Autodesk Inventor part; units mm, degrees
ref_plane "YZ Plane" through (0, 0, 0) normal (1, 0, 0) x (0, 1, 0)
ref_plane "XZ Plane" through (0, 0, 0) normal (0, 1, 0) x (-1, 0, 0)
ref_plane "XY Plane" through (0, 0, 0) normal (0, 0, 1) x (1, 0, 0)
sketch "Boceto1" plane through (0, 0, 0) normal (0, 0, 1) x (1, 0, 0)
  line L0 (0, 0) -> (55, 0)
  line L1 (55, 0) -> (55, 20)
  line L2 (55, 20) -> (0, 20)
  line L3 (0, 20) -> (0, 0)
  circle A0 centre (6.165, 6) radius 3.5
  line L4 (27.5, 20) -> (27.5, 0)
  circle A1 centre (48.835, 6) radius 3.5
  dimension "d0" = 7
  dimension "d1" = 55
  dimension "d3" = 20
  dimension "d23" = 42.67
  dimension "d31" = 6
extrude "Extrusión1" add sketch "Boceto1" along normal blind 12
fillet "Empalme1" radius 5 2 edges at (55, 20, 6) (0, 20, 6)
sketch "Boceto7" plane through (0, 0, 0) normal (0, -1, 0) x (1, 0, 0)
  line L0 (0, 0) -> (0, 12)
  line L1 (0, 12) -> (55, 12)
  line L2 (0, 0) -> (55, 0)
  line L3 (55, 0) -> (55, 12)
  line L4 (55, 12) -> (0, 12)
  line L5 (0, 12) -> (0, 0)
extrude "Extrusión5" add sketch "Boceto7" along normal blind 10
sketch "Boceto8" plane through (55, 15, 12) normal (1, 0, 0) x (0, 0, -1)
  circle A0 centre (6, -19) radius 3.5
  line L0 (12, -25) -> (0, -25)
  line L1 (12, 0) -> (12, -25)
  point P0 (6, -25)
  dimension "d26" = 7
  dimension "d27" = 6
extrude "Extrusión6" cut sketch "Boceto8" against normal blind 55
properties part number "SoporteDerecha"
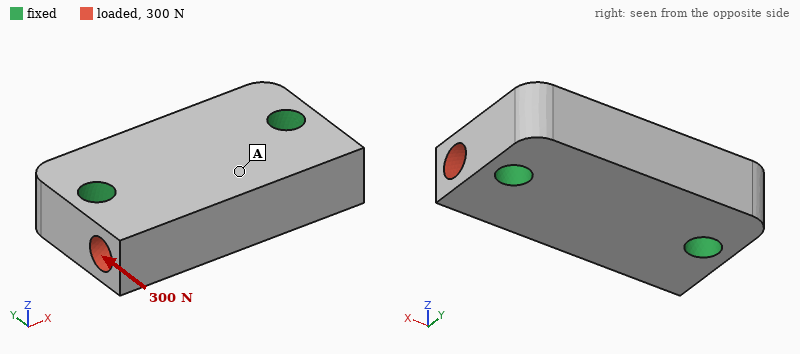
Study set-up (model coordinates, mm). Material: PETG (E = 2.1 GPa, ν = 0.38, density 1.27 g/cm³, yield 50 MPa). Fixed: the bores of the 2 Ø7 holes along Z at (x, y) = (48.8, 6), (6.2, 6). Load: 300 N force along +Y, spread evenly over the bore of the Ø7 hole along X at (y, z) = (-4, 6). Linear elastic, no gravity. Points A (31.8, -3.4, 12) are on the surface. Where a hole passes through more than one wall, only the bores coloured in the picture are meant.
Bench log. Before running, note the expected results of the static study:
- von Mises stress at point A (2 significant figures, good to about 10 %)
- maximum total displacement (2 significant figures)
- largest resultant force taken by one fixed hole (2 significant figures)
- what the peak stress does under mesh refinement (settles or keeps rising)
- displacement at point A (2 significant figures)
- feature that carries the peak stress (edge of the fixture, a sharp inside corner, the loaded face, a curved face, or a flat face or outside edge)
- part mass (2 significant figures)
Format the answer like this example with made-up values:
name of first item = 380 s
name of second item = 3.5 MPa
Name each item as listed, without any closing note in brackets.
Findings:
von Mises stress at point A = 0.35 MPa
maximum total displacement = 12 µm
largest resultant force taken by one fixed hole = 150 N
what the peak stress does under mesh refinement = keeps rising
displacement at point A = 9.1 µm
feature that carries the peak stress = edge of the fixture
part mass = 21 g
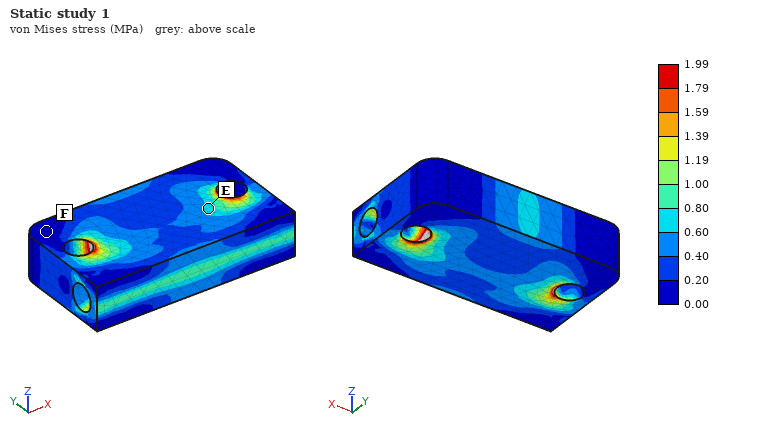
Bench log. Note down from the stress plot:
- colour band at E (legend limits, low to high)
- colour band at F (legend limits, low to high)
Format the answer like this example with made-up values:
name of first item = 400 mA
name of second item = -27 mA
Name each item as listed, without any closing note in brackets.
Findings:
colour band at E = 0.60 to 0.80 MPa
colour band at F = 0.00 to 0.20 MPa
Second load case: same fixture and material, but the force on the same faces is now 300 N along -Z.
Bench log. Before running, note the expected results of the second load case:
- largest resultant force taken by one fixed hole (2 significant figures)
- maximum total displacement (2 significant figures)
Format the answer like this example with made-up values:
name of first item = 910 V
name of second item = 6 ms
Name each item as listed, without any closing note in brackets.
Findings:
largest resultant force taken by one fixed hole = 150 N
maximum total displacement = 55 µm
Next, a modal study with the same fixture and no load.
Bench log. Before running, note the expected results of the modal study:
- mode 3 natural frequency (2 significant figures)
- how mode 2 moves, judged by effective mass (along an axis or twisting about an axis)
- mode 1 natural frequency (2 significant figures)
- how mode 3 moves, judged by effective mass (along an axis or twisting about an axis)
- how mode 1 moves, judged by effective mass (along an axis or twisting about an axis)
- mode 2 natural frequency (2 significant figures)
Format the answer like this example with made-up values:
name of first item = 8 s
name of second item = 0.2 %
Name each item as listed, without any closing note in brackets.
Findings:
mode 3 natural frequency = 7000 Hz
how mode 2 moves, judged by effective mass = along Z
mode 1 natural frequency = 5000 Hz
how mode 3 moves, judged by effective mass = along Y
how mode 1 moves, judged by effective mass = along Z
mode 2 natural frequency = 5800 Hz
